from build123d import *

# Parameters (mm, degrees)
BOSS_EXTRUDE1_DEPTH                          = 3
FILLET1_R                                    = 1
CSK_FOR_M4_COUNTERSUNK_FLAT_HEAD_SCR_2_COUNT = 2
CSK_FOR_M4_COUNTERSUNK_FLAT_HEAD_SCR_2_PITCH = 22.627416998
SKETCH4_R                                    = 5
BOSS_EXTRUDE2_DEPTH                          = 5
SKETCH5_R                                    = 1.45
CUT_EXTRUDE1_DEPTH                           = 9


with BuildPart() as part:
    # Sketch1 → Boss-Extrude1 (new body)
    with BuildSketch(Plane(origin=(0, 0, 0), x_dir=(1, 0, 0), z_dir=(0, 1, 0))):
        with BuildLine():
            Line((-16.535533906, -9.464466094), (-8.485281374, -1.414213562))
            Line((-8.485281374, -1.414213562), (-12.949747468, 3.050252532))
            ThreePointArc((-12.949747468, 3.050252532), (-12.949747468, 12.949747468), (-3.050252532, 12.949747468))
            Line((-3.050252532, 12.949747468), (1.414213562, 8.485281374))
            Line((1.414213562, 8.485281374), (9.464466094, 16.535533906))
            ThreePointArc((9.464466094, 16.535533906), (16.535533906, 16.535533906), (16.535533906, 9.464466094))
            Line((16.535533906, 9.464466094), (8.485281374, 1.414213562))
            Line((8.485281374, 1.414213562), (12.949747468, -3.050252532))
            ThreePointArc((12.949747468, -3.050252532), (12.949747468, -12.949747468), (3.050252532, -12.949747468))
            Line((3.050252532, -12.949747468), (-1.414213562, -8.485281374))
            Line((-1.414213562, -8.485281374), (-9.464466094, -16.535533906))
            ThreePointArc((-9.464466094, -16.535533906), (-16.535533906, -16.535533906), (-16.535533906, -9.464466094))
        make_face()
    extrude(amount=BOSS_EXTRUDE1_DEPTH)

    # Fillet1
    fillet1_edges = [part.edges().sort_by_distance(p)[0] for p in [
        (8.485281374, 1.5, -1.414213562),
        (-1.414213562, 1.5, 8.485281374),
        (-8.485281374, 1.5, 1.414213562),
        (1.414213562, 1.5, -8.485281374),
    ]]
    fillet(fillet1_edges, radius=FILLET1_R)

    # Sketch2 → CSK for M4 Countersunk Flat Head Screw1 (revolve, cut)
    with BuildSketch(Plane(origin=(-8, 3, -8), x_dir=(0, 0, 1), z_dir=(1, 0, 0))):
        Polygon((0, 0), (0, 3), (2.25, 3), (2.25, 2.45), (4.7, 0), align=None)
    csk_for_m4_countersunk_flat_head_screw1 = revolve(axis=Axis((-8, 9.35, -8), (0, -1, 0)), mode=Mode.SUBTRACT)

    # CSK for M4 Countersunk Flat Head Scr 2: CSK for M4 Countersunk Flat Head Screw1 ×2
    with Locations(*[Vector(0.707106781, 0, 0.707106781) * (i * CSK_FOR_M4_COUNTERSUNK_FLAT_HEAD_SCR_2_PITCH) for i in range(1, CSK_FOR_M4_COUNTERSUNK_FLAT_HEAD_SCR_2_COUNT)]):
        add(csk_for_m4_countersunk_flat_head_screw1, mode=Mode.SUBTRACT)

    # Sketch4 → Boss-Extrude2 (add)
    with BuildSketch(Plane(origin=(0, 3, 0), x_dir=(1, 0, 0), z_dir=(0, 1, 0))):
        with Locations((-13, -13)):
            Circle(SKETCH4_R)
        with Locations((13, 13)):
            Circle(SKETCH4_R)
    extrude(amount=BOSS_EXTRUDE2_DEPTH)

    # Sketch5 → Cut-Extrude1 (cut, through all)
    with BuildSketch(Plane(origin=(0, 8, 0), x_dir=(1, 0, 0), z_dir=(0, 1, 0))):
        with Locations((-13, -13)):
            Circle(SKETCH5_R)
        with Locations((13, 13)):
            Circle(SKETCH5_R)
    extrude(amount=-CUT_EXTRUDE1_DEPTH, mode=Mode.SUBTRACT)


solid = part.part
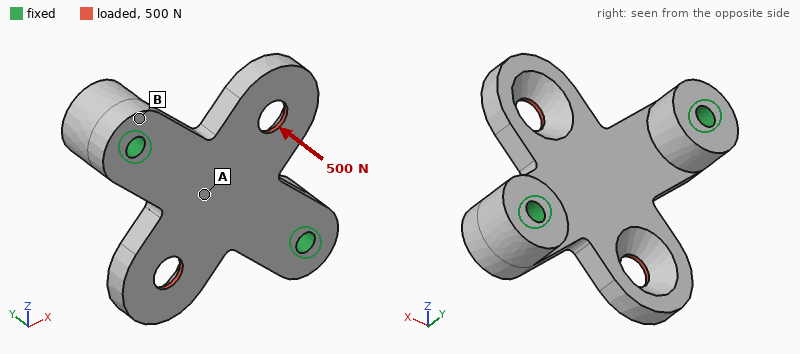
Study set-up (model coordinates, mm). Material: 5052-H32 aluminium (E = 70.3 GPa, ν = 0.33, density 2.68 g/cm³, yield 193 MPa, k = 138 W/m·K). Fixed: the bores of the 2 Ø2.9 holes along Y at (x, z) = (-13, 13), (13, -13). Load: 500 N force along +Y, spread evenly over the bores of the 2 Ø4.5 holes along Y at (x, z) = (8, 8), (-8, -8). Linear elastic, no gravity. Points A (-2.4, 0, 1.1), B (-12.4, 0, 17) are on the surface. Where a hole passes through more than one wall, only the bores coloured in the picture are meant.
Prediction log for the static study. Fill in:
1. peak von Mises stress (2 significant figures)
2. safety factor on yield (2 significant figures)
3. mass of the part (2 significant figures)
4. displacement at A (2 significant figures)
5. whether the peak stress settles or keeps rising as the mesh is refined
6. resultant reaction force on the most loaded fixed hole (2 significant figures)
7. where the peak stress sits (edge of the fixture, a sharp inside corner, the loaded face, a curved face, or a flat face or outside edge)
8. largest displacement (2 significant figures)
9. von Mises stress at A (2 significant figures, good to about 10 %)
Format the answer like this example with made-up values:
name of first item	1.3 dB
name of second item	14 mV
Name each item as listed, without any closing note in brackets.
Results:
peak von Mises stress	150 MPa
safety factor on yield	1.3
mass of the part	7.5 g
displacement at A	0.038 mm
whether the peak stress settles or keeps rising as the mesh is refined	settles
resultant reaction force on the most loaded fixed hole	280 N
where the peak stress sits	a curved face
largest displacement	0.14 mm
von Mises stress at A	99 MPa
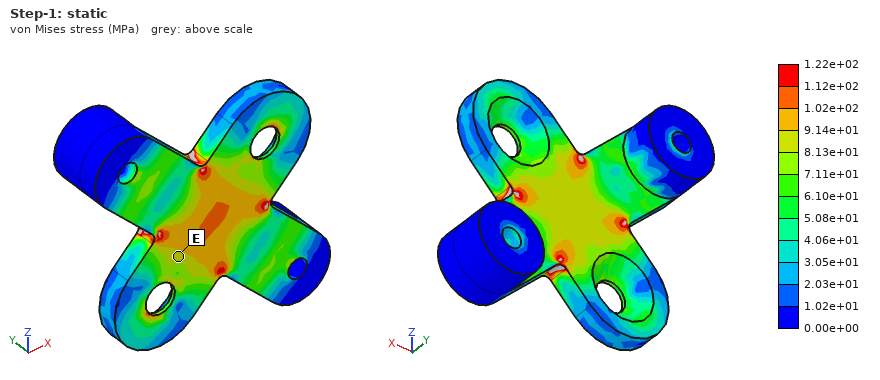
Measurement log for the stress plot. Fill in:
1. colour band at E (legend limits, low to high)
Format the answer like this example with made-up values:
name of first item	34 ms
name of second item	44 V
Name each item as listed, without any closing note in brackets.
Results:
colour band at E	8.13e+01 to 9.14e+01 MPa
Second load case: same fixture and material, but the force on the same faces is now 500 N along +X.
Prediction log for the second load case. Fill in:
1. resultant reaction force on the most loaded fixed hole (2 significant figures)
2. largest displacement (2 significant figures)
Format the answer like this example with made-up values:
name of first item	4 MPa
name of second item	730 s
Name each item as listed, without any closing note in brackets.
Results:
resultant reaction force on the most loaded fixed hole	250 N
largest displacement	32 µm
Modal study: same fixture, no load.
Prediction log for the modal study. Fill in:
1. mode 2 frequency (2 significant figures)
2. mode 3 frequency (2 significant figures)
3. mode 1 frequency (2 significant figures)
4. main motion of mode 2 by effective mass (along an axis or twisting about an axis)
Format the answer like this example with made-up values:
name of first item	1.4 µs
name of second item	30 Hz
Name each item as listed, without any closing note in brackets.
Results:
mode 2 frequency	7800 Hz
mode 3 frequency	18 kHz
mode 1 frequency	5700 Hz
main motion of mode 2 by effective mass	along Y
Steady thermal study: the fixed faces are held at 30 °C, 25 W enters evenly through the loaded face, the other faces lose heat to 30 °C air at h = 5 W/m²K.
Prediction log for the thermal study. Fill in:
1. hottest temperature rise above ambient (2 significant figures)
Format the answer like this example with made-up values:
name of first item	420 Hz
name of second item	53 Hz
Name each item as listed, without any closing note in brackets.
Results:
hottest temperature rise above ambient	68 K
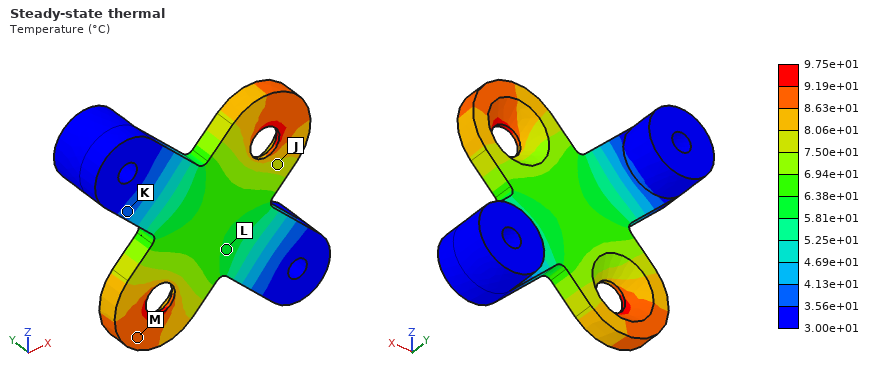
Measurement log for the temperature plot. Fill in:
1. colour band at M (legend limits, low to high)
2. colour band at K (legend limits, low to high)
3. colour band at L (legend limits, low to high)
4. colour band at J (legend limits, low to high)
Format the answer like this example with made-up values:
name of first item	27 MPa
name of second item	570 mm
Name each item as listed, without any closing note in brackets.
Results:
colour band at M	8.63e+01 to 9.19e+01 °C
colour band at K	3.56e+01 to 4.13e+01 °C
colour band at L	5.81e+01 to 6.38e+01 °C
colour band at J	7.50e+01 to 8.06e+01 °C
